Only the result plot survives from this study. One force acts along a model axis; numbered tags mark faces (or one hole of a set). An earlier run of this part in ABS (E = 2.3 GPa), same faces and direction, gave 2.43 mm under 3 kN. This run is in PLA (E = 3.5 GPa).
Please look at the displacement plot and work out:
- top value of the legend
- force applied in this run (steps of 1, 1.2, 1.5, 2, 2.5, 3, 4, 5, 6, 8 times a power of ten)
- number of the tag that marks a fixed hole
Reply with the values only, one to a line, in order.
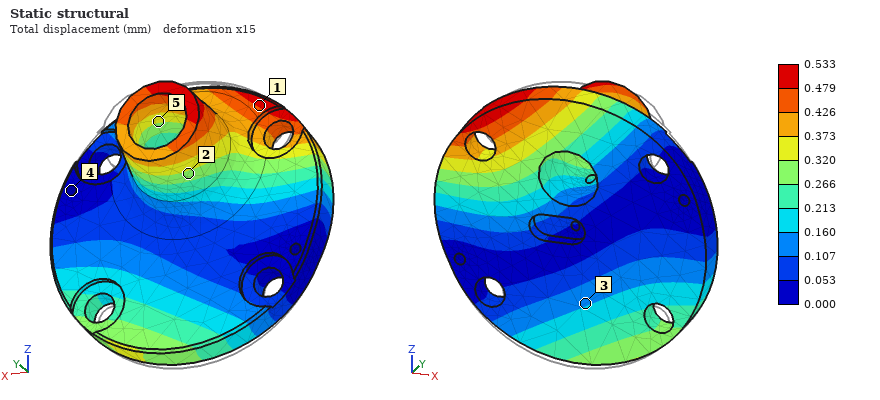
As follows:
0.533 mm
1 kN
4
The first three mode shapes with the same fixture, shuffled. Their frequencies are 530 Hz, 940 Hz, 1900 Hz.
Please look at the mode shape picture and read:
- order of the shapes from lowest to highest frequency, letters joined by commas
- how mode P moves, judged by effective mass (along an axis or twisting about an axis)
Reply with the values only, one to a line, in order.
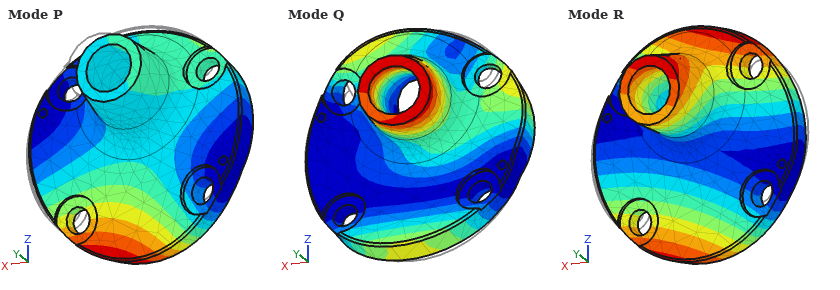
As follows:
R, P, Q
along Y
